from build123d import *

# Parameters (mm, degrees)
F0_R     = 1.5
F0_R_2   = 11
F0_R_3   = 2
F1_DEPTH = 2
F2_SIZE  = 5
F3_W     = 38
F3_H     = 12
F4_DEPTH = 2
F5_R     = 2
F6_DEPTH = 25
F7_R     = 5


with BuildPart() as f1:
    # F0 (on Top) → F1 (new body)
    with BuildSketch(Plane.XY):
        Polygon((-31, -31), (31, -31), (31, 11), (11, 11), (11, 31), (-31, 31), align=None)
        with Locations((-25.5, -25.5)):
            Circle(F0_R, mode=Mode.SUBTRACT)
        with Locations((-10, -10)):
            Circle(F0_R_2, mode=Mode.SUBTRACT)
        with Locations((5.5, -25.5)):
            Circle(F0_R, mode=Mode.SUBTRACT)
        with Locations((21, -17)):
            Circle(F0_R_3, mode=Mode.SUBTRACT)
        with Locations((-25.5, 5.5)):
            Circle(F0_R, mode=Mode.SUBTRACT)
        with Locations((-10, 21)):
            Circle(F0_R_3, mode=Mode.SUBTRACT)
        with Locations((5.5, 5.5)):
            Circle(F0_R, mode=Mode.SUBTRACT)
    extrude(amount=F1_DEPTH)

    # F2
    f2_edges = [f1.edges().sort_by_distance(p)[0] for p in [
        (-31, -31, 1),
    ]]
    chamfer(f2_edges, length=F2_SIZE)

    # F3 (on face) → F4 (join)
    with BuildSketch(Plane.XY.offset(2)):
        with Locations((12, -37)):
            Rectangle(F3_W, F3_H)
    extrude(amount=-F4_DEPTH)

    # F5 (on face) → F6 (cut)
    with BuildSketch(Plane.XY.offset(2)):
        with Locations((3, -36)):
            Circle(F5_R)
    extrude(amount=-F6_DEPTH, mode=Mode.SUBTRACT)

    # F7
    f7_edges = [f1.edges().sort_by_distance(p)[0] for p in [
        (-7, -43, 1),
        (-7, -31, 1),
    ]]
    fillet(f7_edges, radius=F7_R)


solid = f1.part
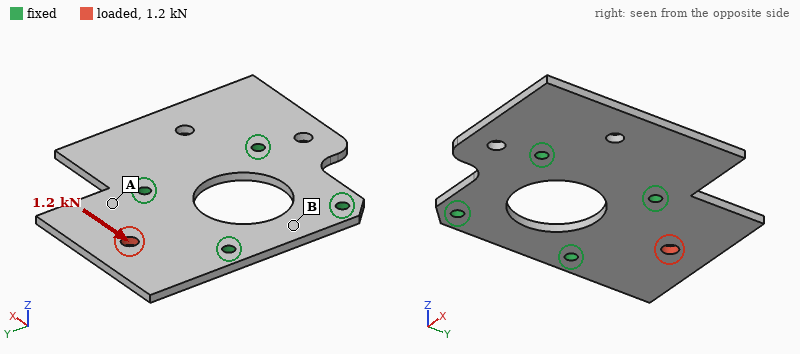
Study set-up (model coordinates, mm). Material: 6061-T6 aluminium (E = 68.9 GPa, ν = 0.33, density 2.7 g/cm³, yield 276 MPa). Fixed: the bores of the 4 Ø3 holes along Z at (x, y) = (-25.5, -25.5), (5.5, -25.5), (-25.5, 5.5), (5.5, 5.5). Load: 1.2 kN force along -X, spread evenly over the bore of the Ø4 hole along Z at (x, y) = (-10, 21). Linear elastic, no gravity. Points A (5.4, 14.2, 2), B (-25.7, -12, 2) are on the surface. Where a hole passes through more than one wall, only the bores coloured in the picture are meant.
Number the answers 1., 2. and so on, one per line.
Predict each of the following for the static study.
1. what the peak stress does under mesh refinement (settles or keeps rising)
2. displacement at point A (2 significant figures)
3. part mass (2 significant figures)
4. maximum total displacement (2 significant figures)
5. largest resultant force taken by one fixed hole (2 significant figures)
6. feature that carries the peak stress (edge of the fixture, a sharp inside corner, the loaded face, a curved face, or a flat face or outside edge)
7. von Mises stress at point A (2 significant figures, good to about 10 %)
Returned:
1. keeps rising
2. 6.7 µm
3. 19 g
4. 17 µm
5. 800 N
6. edge of the fixture
7. 23 MPa
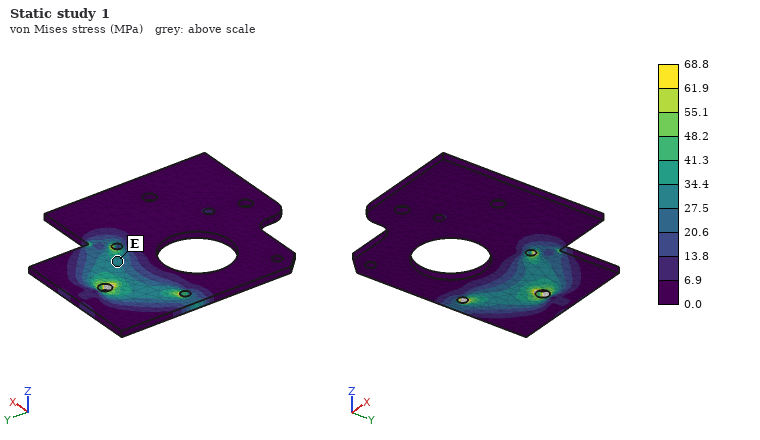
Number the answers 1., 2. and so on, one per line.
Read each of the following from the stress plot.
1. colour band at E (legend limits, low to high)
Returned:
1. 27.5 to 34.4 MPa
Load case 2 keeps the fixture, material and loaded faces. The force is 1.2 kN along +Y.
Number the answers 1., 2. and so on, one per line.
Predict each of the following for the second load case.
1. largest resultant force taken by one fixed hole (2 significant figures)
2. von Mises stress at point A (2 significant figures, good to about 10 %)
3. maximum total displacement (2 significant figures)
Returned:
1. 590 N
2. 16 MPa
3. 12 µm
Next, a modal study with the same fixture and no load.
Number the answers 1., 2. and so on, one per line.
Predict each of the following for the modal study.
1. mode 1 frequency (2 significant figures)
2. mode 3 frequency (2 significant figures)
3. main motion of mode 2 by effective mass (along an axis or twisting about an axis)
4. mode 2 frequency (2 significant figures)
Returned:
1. 2200 Hz
2. 3200 Hz
3. along Z
4. 2400 Hz
